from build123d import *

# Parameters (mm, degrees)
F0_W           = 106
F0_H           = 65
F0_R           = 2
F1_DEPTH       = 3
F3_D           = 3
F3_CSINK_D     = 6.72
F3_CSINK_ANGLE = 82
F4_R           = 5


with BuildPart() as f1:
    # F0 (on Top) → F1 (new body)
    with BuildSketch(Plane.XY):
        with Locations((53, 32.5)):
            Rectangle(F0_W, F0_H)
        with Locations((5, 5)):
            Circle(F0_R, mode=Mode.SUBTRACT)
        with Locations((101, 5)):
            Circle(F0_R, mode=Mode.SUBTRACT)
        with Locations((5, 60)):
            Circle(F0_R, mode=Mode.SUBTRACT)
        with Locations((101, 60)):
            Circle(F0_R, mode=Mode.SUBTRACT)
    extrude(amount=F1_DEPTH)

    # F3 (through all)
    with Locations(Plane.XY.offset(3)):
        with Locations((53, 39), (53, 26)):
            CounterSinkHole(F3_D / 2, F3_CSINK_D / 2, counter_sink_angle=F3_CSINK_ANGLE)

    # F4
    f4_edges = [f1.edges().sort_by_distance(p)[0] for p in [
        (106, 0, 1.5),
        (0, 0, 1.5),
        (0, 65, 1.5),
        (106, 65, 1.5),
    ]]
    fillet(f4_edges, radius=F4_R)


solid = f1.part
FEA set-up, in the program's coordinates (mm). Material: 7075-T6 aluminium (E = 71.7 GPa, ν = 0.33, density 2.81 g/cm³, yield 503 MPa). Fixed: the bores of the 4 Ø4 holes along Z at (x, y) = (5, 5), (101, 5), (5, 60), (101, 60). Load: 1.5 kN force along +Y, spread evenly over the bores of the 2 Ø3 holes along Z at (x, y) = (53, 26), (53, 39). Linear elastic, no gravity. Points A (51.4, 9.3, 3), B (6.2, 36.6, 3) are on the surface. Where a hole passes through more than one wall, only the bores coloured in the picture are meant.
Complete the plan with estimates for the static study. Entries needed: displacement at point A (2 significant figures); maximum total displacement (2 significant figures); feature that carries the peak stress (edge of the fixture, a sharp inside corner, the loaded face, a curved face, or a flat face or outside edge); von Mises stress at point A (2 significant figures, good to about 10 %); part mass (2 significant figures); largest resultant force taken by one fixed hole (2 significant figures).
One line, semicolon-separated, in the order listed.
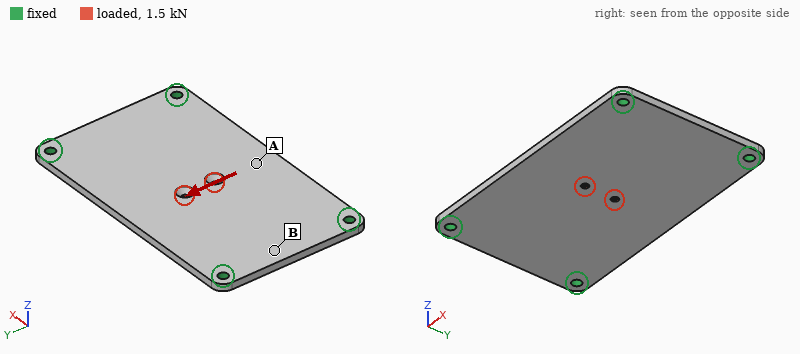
25 µm; 31 µm; the loaded face; 11 MPa; 57 g; 500 N
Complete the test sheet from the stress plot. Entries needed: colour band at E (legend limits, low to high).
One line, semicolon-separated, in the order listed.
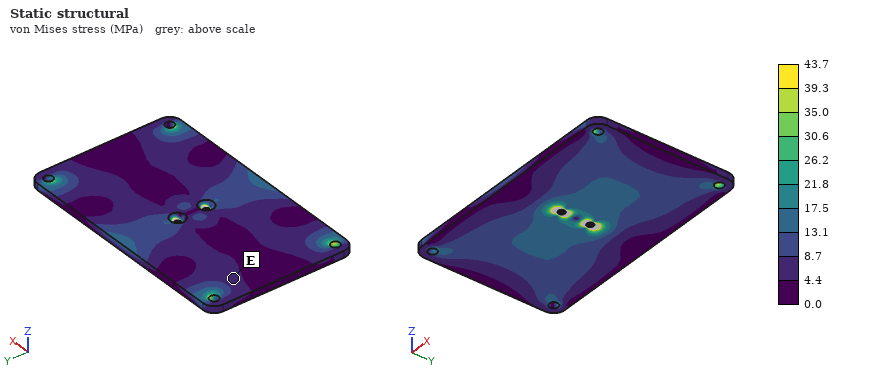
4.4 to 8.7 MPa
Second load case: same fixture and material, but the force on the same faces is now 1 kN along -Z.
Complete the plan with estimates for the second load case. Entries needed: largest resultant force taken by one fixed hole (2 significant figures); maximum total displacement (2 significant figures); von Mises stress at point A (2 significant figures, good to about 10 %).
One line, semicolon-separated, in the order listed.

250 N; 0.66 mm; 110 MPa
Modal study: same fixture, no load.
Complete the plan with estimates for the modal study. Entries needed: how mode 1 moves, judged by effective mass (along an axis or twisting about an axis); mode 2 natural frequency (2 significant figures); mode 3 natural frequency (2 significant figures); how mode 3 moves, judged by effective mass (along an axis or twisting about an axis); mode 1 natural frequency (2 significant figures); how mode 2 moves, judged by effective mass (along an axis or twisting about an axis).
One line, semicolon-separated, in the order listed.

along Z; 2400 Hz; 3800 Hz; twisting about Y; 1400 Hz; twisting about X
